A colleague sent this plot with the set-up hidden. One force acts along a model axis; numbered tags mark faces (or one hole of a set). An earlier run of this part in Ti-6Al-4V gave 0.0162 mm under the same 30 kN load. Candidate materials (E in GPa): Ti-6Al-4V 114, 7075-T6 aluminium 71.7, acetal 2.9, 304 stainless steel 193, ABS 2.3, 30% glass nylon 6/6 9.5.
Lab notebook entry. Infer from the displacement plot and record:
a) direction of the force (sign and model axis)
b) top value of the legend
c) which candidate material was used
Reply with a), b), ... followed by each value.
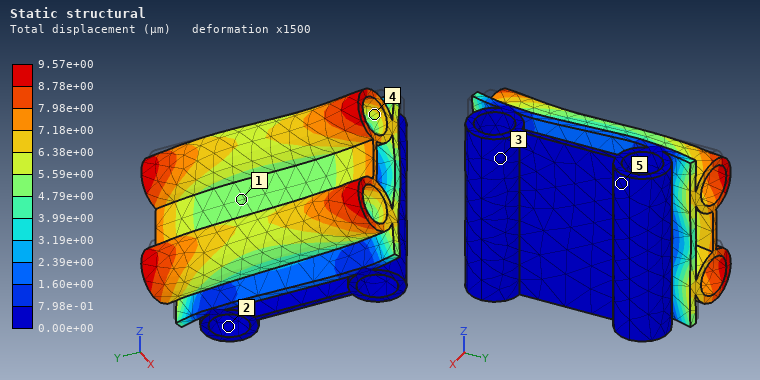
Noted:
a) +Y
b) 9.57e+00 µm
c) 304 stainless steel
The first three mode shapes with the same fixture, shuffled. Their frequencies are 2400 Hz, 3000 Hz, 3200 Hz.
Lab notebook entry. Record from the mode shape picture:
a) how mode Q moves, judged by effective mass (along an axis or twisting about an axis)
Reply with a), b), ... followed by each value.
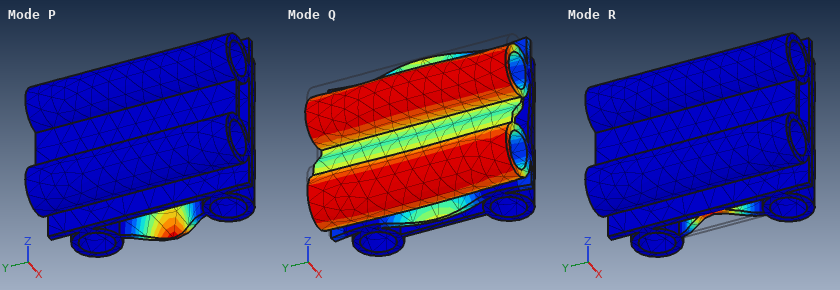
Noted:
a) along Z
